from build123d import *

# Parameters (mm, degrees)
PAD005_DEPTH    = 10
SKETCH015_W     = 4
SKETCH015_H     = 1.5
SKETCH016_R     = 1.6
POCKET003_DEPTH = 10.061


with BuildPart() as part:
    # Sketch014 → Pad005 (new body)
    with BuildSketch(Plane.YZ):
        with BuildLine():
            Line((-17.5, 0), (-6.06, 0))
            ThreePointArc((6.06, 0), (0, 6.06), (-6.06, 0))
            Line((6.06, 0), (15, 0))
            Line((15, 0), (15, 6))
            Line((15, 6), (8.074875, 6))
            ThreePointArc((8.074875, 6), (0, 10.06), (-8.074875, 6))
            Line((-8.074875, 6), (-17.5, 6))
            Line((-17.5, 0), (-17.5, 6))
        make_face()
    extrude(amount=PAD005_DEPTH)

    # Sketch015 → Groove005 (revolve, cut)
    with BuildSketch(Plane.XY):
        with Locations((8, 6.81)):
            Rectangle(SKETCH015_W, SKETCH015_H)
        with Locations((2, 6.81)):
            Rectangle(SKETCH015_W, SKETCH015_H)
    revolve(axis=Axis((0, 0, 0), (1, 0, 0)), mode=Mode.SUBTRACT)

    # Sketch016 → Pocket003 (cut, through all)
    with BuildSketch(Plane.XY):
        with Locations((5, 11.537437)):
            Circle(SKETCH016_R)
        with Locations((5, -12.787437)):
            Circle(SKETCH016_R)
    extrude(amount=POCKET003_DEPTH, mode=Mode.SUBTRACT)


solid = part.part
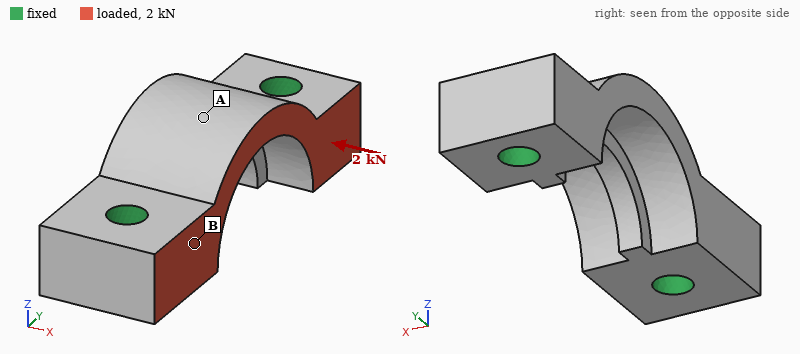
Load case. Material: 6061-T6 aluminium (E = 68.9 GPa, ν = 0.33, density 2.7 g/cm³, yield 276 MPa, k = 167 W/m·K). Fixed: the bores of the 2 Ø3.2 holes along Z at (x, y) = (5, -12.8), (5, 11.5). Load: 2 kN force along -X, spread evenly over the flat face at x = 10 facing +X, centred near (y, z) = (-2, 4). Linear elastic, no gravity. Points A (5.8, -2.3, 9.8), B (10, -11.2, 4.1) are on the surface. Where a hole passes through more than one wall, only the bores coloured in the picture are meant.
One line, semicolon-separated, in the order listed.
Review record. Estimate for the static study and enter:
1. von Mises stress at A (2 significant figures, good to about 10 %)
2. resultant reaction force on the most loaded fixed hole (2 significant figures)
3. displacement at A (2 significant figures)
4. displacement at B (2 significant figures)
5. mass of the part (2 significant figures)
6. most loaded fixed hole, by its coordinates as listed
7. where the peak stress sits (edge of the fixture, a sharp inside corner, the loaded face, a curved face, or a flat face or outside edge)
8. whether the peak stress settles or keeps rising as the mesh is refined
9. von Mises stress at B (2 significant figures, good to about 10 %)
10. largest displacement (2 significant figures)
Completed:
15 MPa; 1.1 kN; 12 µm; 3.1 µm; 4.0 g; (5, -12.8); edge of the fixture; keeps rising; 33 MPa; 15 µm
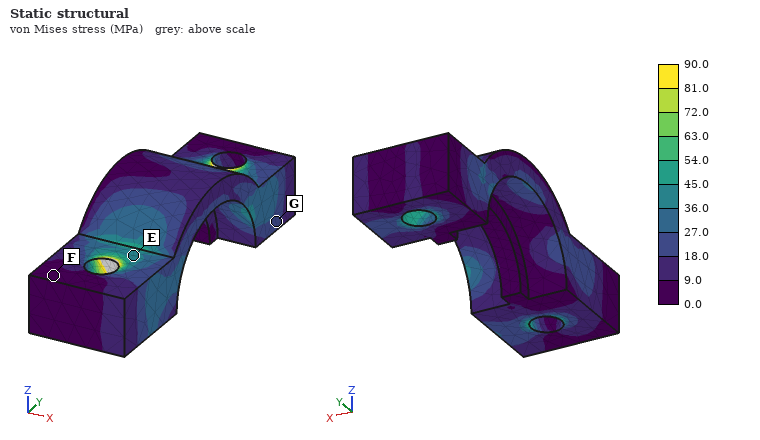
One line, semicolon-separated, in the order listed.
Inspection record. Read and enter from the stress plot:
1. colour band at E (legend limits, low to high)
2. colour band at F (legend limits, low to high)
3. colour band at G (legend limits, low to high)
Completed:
36.0 to 45.0 MPa; 0.0 to 9.0 MPa; 18.0 to 27.0 MPa
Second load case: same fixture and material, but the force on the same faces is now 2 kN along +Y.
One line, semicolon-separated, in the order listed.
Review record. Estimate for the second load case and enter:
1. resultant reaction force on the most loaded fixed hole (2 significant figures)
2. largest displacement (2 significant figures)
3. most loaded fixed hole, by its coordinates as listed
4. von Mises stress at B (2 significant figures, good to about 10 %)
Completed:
1.1 kN; 8.4 µm; (5, -12.8); 25 MPa
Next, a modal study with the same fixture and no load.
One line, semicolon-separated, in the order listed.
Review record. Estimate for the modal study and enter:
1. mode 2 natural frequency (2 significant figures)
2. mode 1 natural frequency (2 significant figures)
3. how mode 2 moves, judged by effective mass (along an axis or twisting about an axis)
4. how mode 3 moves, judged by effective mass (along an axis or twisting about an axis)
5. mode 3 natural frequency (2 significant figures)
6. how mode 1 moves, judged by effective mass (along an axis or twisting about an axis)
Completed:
57 kHz; 34 kHz; along Z; along Y; 66 kHz; along X
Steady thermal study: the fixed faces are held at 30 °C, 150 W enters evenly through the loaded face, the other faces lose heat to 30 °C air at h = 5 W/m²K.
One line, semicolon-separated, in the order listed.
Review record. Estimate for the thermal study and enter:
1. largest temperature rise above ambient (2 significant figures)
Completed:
61 K
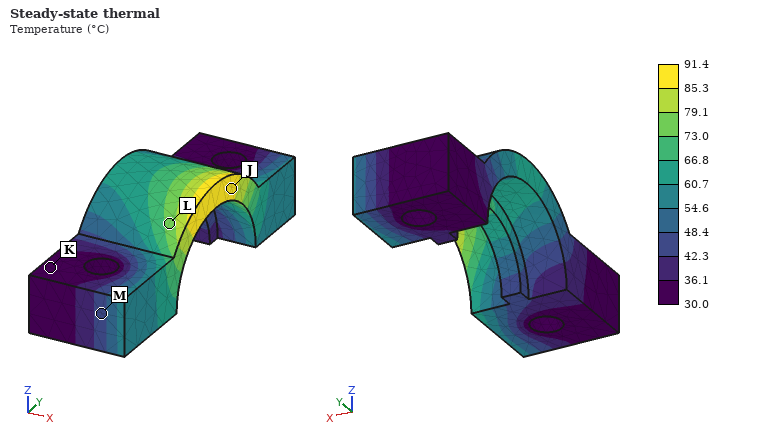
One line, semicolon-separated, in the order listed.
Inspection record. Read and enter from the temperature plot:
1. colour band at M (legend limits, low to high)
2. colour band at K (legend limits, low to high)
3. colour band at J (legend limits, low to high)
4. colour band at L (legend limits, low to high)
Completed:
42.3 to 48.4 °C; 30.0 to 36.1 °C; 85.3 to 91.4 °C; 73.0 to 79.1 °C
